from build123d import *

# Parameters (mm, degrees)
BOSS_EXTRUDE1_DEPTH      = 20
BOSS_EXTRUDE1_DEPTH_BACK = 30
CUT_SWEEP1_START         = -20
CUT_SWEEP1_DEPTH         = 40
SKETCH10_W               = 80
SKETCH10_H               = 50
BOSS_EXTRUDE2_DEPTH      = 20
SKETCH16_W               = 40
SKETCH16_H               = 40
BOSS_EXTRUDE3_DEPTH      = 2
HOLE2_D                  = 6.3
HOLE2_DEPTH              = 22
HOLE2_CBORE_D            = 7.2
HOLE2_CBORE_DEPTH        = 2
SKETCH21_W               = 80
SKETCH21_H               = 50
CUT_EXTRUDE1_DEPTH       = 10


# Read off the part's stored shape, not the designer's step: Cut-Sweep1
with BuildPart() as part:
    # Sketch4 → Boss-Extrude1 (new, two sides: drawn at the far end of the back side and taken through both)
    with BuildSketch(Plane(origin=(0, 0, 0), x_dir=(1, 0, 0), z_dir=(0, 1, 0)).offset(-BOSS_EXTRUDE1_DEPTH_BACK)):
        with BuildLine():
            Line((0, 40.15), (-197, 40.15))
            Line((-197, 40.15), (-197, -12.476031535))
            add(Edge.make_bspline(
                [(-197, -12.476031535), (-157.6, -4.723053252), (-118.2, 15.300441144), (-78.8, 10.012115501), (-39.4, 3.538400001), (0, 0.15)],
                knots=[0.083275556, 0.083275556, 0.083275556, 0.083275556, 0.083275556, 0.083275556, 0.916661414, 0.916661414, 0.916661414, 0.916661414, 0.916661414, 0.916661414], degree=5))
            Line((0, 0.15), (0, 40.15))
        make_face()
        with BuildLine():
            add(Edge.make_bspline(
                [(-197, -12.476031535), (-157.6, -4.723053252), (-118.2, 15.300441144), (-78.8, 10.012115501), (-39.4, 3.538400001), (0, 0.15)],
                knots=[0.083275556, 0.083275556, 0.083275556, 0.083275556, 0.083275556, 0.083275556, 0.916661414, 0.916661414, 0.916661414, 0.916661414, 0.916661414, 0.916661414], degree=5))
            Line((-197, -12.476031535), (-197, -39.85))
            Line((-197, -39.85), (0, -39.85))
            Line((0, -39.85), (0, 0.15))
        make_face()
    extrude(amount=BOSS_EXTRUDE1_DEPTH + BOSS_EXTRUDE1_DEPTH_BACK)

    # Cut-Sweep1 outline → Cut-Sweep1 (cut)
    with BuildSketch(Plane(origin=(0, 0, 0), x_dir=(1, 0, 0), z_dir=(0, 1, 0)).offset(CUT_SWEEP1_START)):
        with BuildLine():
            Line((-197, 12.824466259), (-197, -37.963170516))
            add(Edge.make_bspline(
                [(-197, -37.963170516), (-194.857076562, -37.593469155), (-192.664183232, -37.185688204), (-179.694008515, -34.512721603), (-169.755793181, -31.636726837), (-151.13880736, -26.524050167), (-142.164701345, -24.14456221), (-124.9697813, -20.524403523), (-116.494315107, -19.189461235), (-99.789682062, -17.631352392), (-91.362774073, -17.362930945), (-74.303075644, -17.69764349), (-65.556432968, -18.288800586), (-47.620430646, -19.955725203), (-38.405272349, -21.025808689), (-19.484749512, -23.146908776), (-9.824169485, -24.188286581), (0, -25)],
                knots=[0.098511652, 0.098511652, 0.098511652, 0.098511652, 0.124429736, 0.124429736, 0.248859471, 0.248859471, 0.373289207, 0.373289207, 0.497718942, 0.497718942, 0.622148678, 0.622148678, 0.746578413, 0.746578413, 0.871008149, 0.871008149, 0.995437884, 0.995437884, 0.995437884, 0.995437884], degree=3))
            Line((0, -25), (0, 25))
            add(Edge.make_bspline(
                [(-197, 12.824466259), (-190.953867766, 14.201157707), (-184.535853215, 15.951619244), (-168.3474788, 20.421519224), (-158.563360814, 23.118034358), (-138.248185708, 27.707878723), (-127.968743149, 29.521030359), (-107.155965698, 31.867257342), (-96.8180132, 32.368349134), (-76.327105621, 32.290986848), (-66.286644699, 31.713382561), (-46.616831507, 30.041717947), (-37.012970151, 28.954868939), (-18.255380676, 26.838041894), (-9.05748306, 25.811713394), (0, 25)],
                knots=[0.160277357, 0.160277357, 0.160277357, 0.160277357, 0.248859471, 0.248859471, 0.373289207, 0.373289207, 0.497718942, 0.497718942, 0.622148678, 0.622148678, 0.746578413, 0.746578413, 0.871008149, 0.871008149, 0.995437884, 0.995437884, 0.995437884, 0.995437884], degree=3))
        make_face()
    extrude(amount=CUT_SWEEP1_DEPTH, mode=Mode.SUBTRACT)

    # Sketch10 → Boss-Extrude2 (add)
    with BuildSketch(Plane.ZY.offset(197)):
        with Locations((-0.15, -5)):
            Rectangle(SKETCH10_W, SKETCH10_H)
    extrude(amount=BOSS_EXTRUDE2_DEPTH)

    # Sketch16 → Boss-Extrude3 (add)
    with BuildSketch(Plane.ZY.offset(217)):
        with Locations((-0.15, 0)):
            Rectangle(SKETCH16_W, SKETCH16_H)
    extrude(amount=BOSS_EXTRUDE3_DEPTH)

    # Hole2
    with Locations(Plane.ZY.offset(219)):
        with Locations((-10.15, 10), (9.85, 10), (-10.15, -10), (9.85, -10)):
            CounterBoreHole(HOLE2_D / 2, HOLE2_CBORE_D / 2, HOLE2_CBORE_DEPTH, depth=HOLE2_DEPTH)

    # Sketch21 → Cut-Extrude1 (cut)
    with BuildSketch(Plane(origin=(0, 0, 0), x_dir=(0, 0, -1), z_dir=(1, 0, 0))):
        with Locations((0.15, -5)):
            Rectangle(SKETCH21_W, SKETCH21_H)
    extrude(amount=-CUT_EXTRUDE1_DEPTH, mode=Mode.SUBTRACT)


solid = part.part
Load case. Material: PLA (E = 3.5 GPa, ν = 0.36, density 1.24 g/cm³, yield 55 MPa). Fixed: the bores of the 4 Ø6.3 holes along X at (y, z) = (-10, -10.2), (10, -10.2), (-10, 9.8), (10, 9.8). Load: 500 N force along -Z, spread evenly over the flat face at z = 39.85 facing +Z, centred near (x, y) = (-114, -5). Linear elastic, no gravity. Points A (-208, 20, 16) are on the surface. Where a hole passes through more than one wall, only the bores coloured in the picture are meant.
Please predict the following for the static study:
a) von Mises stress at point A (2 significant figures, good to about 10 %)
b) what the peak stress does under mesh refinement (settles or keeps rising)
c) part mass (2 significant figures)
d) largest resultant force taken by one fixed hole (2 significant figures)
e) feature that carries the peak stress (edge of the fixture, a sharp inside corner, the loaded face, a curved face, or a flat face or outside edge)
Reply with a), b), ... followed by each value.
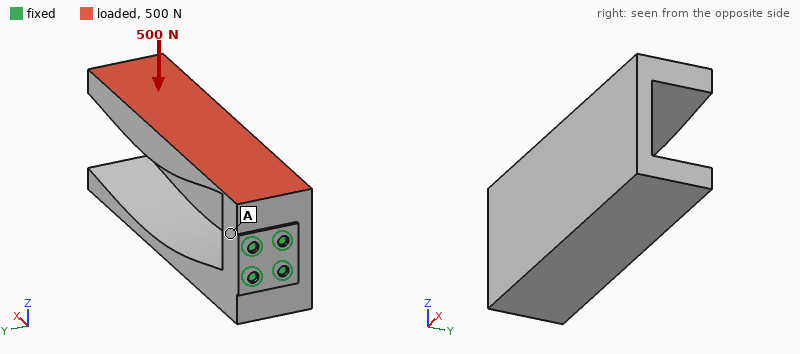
a) 1.4 MPa
b) keeps rising
c) 560 g
d) 820 N
e) edge of the fixture
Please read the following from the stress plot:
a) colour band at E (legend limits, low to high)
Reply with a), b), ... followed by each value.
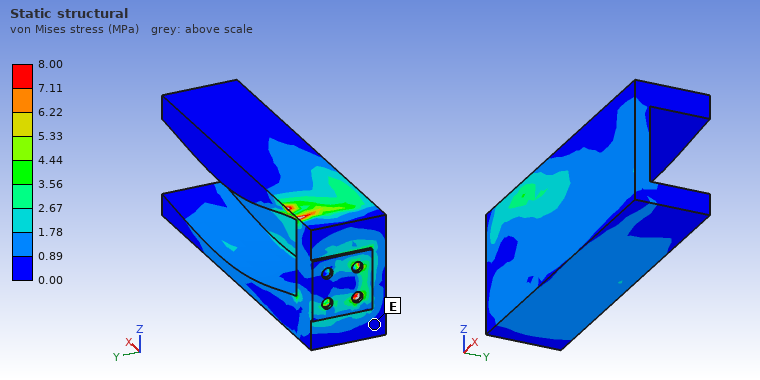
a) 0.00 to 0.89 MPa
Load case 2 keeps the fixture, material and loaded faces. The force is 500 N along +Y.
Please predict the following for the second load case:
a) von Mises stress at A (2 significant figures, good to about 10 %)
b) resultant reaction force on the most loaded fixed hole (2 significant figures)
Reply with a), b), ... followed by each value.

a) 4.5 MPa
b) 860 N
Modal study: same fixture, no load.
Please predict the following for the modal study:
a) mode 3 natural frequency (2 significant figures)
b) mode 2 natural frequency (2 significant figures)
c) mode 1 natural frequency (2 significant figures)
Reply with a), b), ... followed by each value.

a) 510 Hz
b) 250 Hz
c) 190 Hz
